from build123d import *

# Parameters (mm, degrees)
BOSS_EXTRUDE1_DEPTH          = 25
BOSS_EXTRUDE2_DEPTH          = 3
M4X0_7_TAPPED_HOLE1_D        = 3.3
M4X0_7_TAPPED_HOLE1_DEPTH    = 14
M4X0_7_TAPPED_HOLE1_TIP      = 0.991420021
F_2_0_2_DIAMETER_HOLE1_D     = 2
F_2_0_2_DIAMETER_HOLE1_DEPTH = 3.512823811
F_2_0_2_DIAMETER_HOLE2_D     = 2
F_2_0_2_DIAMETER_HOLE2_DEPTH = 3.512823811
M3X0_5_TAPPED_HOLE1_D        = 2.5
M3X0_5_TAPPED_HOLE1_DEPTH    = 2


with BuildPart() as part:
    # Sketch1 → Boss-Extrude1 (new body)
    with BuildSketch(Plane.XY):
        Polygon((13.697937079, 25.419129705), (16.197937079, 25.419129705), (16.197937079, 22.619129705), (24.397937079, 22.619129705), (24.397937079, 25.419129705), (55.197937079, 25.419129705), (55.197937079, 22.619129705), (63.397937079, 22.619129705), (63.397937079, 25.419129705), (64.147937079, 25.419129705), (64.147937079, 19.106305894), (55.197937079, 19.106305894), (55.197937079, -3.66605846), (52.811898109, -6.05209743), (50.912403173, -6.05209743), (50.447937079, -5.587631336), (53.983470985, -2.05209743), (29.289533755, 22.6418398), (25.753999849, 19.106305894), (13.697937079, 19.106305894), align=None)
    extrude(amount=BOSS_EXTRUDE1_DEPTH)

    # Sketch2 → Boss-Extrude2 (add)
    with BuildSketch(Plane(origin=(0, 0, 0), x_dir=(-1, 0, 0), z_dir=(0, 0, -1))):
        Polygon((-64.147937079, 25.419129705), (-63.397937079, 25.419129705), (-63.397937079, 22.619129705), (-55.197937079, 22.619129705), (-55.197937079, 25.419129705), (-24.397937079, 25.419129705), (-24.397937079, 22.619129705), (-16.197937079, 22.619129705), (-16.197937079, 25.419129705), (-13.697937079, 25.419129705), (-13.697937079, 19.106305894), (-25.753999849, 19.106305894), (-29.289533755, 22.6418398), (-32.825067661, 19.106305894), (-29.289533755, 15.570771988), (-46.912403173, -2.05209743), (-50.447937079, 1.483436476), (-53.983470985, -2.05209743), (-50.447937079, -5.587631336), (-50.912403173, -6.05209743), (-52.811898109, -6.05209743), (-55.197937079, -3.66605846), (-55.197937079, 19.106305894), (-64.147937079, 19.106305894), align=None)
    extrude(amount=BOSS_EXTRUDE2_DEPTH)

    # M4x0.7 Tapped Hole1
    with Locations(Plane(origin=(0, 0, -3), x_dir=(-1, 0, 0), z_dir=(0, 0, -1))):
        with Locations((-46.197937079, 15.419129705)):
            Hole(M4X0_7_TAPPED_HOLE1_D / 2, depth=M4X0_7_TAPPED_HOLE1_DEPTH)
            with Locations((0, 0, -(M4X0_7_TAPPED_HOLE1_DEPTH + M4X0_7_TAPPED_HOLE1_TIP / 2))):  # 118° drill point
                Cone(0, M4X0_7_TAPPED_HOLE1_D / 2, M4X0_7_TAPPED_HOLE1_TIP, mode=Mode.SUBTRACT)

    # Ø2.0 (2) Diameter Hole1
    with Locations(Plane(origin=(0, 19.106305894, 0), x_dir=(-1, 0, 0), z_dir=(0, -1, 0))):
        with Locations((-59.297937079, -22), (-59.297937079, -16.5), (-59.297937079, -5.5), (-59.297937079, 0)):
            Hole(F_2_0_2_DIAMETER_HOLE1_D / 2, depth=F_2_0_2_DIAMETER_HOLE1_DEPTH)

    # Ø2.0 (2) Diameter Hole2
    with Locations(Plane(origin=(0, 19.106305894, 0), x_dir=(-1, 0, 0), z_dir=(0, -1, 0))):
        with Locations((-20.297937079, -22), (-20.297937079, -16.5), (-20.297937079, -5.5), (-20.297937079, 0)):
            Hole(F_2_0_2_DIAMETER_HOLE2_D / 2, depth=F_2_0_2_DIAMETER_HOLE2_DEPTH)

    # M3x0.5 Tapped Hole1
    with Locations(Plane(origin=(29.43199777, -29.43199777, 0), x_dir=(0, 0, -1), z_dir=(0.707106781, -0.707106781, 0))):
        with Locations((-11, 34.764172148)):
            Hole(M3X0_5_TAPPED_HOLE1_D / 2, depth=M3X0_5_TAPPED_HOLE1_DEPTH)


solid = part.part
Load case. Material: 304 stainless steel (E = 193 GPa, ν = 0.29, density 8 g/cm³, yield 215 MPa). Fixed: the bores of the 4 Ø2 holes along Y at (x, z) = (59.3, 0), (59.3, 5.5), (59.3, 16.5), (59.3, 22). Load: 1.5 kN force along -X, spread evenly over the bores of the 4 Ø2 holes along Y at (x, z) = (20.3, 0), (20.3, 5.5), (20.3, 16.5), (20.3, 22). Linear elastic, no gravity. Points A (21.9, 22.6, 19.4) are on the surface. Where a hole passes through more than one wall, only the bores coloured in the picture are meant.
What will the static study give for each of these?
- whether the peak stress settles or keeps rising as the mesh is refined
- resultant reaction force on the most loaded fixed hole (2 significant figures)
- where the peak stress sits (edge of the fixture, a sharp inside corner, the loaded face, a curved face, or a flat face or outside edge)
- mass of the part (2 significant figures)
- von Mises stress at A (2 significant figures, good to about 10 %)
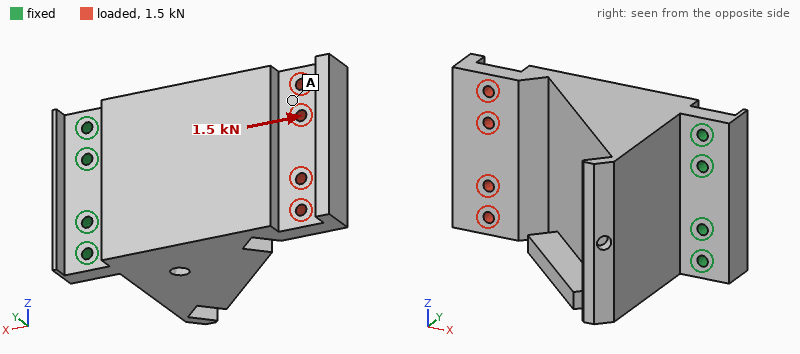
keeps rising
410 N
a sharp inside corner
120 g
14 MPa
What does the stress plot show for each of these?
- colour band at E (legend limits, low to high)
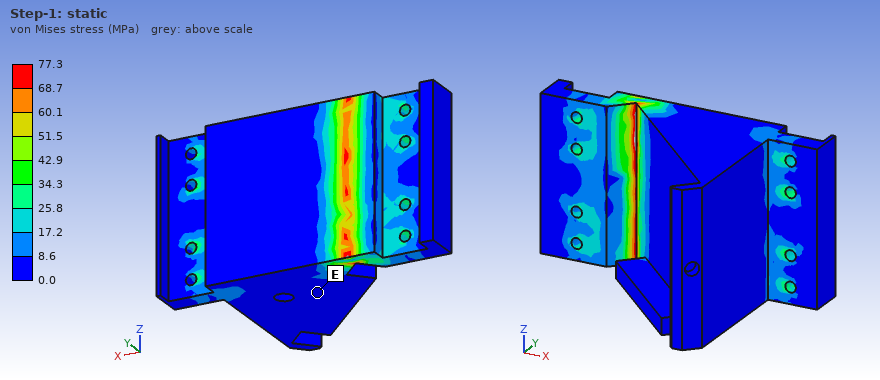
0.0 to 8.6 MPa
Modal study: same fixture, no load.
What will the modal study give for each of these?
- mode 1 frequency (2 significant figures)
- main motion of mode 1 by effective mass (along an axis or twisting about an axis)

1500 Hz
along Y
